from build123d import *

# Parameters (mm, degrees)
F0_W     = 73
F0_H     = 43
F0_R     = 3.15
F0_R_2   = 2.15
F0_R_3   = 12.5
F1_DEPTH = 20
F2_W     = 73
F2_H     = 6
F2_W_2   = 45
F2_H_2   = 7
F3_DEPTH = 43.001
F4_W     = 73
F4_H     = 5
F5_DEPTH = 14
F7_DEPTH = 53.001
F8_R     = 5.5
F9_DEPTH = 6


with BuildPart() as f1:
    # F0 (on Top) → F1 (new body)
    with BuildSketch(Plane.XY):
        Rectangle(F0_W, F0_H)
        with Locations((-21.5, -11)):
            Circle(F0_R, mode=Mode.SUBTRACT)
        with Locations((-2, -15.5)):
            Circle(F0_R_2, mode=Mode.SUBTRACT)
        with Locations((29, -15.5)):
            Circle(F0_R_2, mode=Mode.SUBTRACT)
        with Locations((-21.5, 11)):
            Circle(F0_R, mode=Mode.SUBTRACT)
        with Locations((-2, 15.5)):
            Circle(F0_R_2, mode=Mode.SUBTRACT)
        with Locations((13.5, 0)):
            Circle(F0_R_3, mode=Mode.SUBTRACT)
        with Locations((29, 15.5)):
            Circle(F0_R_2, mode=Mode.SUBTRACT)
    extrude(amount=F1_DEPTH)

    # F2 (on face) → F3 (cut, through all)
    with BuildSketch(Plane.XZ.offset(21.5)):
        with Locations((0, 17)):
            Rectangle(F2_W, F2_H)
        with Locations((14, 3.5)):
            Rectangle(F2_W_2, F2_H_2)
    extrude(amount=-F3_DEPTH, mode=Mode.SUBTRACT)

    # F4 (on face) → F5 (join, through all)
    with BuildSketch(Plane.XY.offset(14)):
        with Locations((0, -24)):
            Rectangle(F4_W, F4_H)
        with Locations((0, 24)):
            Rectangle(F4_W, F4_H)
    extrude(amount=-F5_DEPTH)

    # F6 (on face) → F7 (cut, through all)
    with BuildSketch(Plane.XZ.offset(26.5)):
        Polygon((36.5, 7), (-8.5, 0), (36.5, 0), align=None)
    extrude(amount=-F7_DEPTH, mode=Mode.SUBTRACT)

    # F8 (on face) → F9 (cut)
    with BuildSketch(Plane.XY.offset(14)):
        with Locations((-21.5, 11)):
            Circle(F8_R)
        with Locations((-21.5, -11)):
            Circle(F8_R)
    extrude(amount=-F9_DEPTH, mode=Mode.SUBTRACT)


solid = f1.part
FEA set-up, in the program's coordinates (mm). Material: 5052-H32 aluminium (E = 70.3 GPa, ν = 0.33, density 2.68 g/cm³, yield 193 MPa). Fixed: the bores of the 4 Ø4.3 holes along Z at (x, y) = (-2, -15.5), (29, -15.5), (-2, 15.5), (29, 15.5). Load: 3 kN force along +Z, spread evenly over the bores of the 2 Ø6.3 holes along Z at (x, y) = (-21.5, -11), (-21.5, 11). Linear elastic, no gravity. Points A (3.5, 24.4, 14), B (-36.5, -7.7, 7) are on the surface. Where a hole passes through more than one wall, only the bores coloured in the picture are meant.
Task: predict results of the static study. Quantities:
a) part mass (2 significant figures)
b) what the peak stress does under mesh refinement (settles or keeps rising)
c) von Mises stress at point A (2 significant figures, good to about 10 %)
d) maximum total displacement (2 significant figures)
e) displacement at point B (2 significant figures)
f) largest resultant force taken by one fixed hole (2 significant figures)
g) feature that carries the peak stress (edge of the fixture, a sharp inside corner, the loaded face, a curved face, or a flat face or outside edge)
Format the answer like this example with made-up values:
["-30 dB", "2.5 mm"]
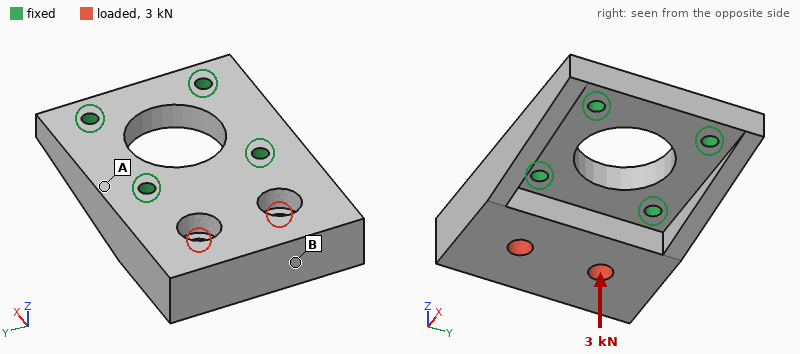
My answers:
["90 g", "keeps rising", "30 MPa", "0.11 mm", "0.11 mm", "2.0 kN", "edge of the fixture"]
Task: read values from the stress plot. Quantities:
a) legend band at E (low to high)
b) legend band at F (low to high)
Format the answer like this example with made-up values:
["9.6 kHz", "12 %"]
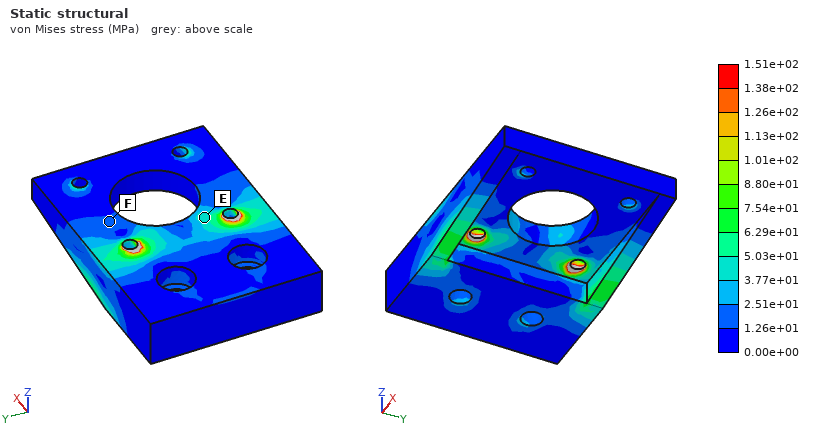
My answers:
["3.77e+01 to 5.03e+01 MPa", "1.26e+01 to 2.51e+01 MPa"]
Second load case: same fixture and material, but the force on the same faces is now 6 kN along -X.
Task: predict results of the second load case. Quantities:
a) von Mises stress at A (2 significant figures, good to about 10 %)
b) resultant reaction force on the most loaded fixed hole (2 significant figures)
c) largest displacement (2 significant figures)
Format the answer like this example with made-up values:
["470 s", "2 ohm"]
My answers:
["14 MPa", "2.6 kN", "81 µm"]
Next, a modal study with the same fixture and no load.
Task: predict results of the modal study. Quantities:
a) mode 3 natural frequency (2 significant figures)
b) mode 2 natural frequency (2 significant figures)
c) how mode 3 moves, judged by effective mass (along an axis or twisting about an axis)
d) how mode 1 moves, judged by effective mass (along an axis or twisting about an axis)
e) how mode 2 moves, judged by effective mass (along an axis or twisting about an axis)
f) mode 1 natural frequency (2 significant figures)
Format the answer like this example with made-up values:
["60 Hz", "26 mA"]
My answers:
["12 kHz", "8900 Hz", "along Y", "along Z", "twisting about X", "4200 Hz"]
